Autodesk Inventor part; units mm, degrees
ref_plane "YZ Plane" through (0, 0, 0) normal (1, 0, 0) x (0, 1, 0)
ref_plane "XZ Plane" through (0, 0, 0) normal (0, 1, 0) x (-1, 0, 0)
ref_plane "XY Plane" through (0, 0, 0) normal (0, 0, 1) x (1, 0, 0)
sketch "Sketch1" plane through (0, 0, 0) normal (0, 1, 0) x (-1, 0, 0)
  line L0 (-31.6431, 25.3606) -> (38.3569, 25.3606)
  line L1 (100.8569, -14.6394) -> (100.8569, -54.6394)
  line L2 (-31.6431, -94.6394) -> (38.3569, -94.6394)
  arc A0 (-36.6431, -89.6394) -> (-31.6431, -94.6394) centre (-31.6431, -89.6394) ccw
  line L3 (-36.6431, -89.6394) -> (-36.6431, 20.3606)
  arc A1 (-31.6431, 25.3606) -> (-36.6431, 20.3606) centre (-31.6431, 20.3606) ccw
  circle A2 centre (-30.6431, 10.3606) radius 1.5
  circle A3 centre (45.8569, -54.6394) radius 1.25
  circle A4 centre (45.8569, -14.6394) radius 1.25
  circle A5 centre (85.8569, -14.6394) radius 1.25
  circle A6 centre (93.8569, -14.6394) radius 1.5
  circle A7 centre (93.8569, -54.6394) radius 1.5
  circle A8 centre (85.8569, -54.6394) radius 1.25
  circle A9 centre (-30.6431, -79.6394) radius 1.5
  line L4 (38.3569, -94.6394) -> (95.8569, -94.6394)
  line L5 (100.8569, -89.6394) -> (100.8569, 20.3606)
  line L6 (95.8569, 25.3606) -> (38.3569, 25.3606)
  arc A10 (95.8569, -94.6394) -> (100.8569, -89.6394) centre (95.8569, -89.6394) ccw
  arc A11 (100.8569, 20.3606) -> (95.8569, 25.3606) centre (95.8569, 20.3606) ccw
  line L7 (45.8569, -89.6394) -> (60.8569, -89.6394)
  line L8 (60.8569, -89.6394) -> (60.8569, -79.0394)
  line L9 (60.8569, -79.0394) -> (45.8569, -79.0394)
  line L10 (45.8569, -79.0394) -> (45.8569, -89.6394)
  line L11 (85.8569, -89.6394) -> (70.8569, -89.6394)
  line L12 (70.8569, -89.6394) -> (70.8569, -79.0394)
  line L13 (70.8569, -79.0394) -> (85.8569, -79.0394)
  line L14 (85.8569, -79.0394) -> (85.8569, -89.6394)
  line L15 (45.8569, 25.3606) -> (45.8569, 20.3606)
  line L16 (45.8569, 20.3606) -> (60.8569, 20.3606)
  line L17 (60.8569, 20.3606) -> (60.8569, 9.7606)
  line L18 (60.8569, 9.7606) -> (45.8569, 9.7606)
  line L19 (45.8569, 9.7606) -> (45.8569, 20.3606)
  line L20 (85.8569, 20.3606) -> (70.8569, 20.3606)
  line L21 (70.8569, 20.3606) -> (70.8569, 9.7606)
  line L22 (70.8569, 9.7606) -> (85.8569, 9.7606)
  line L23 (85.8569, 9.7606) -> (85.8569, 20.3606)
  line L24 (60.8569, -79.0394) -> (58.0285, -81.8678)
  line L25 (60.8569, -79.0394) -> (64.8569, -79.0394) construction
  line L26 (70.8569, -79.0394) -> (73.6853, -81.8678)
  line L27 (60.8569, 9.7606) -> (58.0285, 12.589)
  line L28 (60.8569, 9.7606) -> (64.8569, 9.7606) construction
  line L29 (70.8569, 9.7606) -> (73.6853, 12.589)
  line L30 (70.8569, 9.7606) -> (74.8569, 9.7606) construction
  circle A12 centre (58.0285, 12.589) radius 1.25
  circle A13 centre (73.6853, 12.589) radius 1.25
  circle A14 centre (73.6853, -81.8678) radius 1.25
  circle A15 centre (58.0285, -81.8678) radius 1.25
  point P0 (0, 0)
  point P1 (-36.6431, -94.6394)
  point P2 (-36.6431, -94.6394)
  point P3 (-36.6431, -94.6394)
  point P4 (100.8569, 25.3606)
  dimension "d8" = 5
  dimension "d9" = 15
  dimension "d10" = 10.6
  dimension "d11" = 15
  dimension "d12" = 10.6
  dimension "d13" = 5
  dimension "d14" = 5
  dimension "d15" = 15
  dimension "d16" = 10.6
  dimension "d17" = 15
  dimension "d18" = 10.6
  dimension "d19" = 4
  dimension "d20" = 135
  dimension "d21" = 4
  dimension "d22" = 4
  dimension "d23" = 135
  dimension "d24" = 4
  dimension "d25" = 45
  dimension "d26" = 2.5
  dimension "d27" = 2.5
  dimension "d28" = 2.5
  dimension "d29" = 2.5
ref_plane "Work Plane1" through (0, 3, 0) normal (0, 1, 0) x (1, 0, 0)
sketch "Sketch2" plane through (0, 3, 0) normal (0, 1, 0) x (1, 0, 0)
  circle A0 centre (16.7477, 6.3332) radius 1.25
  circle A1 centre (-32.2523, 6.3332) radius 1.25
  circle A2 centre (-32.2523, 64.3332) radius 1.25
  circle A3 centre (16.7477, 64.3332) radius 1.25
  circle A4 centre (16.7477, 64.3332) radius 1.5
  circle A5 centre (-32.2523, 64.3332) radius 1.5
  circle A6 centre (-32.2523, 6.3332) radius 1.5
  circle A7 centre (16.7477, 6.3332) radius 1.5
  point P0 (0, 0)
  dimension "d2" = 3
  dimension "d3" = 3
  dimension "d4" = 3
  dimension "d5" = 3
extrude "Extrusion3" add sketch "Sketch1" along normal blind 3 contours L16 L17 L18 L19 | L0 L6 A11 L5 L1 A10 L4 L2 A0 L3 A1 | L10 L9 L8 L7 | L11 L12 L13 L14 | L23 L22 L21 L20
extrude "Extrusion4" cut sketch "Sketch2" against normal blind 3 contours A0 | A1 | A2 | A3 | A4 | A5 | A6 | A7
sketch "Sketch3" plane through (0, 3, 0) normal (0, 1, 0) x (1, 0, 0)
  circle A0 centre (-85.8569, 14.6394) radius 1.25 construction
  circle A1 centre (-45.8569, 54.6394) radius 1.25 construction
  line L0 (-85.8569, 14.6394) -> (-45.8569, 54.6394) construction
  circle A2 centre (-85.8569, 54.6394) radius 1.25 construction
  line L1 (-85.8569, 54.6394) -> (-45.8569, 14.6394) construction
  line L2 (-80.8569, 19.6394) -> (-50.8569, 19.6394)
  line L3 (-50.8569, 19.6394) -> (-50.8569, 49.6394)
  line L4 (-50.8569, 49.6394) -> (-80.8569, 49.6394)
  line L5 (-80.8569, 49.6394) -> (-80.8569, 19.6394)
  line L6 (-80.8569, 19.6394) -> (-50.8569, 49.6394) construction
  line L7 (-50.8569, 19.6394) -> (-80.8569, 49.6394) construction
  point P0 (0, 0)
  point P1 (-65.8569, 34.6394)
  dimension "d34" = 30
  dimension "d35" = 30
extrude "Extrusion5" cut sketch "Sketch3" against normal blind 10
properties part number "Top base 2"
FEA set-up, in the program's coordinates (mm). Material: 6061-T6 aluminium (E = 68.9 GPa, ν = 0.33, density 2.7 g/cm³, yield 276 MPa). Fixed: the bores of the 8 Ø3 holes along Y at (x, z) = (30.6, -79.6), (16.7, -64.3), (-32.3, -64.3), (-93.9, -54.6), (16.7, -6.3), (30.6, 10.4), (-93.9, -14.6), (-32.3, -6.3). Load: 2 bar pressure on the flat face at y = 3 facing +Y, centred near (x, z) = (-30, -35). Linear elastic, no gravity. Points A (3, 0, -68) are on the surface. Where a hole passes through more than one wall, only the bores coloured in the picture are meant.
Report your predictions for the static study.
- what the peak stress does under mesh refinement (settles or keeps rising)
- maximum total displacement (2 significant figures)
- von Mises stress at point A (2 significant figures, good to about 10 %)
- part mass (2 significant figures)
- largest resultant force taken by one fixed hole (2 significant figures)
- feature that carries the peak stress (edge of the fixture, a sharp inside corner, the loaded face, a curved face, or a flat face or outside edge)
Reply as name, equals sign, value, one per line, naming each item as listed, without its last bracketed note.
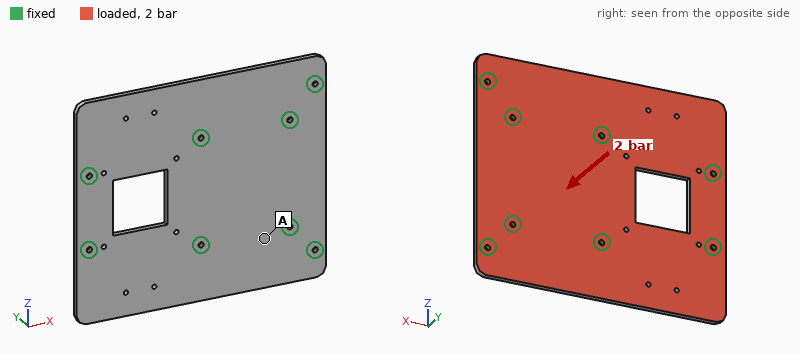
what the peak stress does under mesh refinement = keeps rising
maximum total displacement = 0.47 mm
von Mises stress at point A = 24 MPa
part mass = 130 g
largest resultant force taken by one fixed hole = 700 N
feature that carries the peak stress = edge of the fixture
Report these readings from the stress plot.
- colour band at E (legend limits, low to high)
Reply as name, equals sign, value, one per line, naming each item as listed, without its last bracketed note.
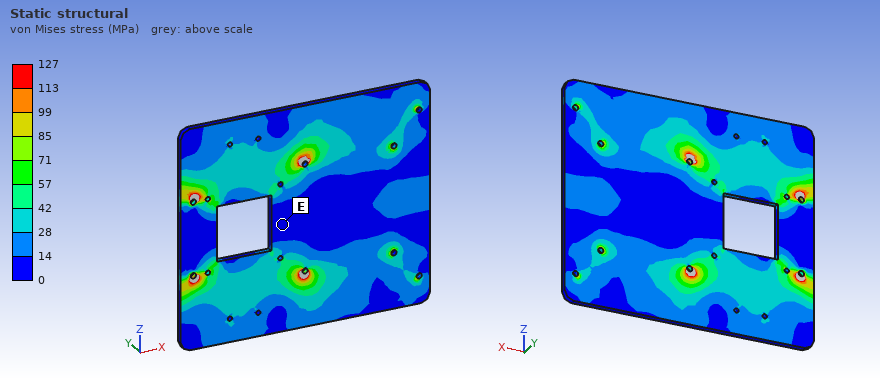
colour band at E = 0 to 14 MPa
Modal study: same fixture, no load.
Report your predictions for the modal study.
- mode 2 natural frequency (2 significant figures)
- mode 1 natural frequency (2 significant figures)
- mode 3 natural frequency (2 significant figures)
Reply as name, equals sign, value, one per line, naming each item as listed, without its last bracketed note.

mode 2 natural frequency = 1500 Hz
mode 1 natural frequency = 1500 Hz
mode 3 natural frequency = 2600 Hz
